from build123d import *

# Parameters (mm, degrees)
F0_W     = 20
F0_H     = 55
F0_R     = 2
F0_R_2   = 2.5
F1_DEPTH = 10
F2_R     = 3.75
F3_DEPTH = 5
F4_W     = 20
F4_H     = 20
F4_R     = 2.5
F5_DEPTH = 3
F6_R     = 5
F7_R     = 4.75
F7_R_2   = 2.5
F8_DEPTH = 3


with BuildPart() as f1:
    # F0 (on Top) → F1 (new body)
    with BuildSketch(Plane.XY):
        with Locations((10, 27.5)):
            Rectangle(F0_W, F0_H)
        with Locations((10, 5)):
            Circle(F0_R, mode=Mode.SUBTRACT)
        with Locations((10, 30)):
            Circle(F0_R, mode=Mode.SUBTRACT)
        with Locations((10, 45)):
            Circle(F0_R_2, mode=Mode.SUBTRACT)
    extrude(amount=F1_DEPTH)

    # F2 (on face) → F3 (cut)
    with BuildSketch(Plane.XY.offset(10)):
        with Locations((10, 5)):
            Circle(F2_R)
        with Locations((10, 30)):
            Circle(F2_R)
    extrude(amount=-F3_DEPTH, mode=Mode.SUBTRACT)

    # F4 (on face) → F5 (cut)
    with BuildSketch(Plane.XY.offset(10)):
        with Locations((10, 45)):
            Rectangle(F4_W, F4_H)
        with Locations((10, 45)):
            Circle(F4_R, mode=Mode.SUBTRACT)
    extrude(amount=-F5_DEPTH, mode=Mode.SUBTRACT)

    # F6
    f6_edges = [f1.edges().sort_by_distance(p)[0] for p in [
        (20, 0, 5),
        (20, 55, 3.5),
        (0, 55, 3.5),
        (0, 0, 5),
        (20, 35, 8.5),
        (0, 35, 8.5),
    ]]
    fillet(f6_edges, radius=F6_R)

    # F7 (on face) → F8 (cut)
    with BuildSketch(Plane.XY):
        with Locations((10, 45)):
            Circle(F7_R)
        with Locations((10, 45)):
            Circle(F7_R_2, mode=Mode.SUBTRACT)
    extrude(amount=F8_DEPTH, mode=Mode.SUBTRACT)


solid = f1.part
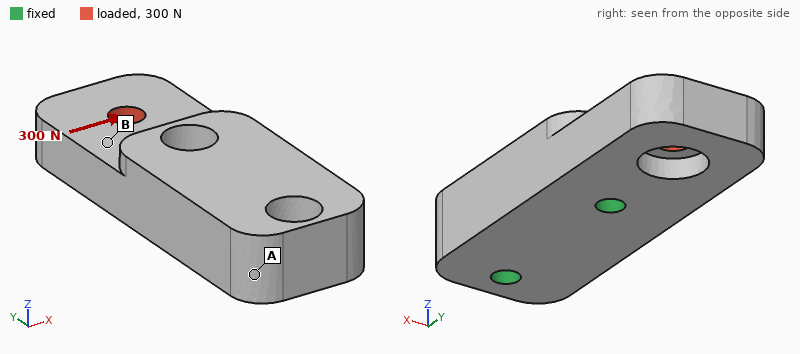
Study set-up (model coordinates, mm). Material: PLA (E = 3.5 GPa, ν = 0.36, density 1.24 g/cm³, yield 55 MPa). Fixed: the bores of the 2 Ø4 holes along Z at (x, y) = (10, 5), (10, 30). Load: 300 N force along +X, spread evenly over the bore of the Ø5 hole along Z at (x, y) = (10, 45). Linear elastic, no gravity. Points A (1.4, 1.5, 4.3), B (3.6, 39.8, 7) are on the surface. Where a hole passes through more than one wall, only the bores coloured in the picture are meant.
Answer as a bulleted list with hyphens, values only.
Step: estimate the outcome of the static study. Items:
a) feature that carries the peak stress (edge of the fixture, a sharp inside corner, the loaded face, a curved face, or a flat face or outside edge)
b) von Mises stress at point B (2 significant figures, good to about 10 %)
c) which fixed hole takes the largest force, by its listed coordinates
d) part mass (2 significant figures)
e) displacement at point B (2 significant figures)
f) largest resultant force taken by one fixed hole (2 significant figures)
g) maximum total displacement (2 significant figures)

- edge of the fixture
- 6.6 MPa
- (10, 30)
- 11 g
- 0.077 mm
- 440 N
- 0.17 mm
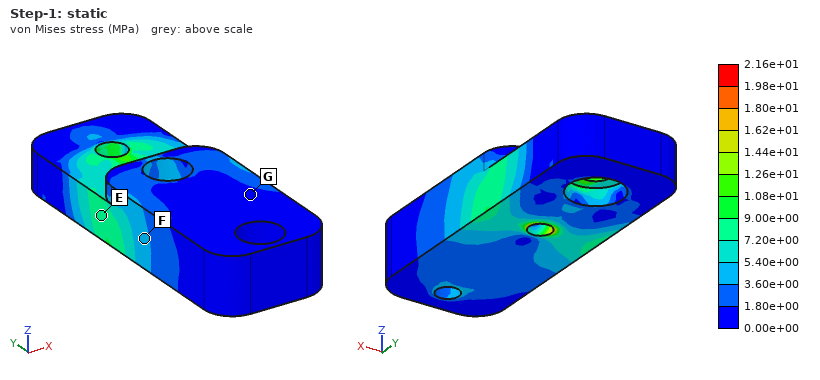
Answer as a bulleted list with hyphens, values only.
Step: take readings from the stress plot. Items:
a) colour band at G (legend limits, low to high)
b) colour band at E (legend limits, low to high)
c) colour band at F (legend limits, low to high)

- 0.00e+00 to 1.80e+00 MPa
- 7.20e+00 to 9.00e+00 MPa
- 3.60e+00 to 5.40e+00 MPa
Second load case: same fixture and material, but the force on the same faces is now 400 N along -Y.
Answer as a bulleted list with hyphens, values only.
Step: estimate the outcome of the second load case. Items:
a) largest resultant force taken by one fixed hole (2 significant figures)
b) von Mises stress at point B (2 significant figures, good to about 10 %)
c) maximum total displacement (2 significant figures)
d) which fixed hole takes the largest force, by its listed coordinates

- 300 N
- 5.8 MPa
- 96 µm
- (10, 30)
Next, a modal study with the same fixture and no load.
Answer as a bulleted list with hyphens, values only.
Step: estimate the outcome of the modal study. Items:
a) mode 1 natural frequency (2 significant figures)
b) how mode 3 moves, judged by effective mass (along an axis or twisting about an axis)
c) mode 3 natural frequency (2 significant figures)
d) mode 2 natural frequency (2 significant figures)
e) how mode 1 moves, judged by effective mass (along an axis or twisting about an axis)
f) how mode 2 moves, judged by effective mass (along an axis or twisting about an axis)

- 2900 Hz
- twisting about Y
- 5100 Hz
- 4600 Hz
- along Z
- along X
